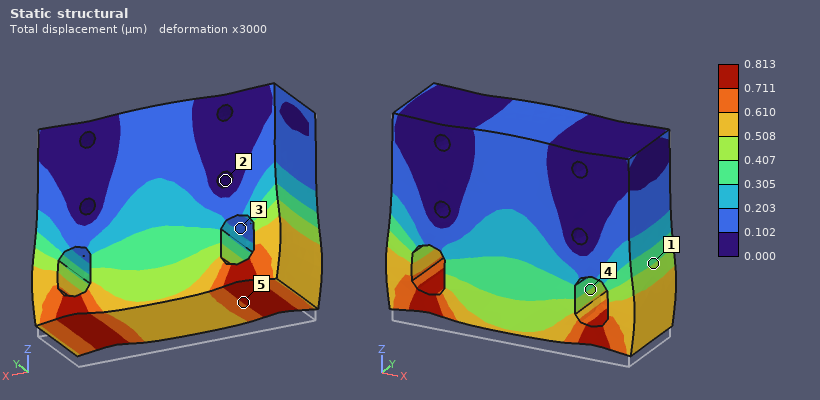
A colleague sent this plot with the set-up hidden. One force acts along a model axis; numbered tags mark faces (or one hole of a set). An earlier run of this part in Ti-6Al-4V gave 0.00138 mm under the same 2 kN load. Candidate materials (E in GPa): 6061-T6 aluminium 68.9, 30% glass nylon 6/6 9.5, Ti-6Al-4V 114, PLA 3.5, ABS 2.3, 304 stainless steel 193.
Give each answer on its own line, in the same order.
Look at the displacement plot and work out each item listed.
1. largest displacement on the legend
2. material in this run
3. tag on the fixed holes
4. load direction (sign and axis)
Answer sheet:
0.813 µm
304 stainless steel
2
+Z
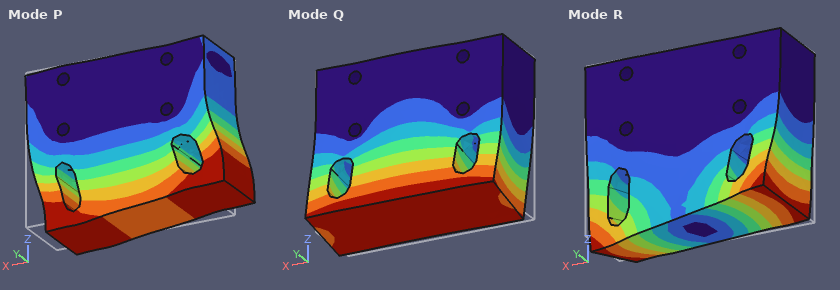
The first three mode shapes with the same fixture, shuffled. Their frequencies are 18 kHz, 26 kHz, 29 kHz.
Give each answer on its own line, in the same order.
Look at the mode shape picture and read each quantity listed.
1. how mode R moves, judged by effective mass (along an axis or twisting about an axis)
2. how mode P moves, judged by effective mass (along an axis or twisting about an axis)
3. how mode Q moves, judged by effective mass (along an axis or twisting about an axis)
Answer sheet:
twisting about Z
along X
along Y
